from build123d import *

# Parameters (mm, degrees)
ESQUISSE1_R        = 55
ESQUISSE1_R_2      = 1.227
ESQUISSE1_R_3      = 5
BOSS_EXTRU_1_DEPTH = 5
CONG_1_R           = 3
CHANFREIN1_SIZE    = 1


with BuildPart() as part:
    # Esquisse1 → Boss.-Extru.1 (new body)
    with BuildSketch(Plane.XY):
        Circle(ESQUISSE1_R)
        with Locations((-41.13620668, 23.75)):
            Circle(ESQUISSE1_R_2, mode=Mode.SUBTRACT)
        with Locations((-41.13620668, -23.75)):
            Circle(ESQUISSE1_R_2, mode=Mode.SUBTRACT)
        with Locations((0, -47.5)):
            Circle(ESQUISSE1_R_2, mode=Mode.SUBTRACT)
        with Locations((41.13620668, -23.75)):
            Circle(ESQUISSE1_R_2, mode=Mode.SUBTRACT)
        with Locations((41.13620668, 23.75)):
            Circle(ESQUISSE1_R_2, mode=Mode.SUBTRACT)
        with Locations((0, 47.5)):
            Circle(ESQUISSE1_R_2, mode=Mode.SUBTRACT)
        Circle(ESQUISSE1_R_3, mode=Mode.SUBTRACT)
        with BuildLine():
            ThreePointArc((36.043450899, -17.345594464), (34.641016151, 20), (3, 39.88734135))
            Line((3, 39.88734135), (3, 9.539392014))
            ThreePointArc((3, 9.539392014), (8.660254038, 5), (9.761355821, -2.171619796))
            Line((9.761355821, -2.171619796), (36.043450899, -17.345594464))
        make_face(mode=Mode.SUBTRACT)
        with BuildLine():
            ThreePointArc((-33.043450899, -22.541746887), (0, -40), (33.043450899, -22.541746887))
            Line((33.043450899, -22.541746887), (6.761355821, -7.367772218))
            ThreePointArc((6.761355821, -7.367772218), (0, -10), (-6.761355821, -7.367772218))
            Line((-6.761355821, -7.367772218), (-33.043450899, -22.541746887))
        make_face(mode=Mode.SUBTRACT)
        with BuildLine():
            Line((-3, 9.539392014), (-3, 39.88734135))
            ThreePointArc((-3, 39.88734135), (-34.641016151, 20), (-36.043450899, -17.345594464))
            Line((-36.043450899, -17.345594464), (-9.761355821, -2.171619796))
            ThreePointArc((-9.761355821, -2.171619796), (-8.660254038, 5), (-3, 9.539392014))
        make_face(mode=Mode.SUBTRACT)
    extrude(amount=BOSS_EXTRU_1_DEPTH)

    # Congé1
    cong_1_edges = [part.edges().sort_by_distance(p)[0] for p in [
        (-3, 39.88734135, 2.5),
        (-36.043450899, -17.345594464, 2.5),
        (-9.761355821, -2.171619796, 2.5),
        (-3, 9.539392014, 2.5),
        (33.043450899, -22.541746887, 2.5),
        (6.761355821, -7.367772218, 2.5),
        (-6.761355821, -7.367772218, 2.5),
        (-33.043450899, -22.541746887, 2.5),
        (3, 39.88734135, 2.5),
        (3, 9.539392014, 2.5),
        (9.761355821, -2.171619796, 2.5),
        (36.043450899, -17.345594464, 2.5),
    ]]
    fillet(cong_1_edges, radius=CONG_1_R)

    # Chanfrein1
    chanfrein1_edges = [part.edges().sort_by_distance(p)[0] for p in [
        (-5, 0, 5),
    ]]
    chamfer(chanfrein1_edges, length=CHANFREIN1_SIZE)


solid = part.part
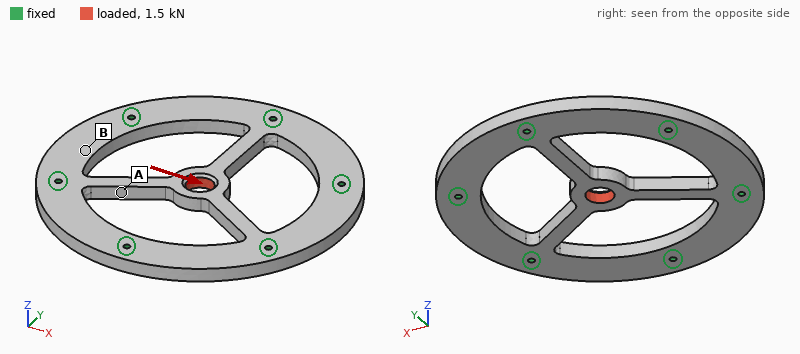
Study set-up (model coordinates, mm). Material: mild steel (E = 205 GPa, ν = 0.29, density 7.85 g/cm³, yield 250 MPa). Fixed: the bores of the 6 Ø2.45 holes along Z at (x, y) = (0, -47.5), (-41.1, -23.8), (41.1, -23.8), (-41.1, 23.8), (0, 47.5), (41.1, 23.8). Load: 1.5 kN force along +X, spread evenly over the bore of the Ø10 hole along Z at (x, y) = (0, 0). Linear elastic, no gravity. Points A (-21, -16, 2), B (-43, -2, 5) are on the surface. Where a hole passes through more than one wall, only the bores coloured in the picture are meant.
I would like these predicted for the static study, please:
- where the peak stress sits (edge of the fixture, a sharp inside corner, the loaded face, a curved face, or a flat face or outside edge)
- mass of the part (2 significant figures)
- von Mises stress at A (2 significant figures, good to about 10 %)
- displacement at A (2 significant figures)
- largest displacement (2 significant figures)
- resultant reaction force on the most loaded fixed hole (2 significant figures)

the loaded face
210 g
24 MPa
2.6 µm
11 µm
790 N
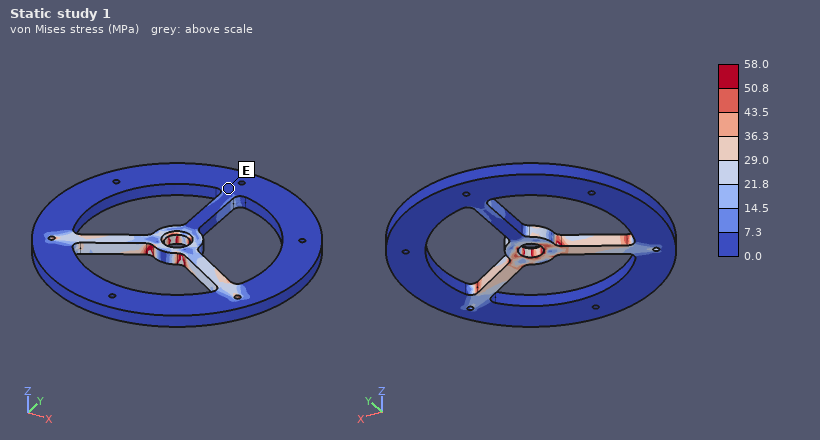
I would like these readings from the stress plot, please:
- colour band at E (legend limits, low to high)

0.0 to 7.3 MPa
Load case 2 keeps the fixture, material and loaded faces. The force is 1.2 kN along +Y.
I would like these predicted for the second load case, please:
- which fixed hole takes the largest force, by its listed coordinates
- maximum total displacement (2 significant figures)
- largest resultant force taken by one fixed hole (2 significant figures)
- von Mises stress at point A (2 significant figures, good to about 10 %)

(0, 47.5)
8.9 µm
730 N
19 MPa
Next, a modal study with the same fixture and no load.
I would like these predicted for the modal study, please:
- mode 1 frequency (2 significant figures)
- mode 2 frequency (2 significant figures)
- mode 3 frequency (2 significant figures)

3300 Hz
7900 Hz
8300 Hz
